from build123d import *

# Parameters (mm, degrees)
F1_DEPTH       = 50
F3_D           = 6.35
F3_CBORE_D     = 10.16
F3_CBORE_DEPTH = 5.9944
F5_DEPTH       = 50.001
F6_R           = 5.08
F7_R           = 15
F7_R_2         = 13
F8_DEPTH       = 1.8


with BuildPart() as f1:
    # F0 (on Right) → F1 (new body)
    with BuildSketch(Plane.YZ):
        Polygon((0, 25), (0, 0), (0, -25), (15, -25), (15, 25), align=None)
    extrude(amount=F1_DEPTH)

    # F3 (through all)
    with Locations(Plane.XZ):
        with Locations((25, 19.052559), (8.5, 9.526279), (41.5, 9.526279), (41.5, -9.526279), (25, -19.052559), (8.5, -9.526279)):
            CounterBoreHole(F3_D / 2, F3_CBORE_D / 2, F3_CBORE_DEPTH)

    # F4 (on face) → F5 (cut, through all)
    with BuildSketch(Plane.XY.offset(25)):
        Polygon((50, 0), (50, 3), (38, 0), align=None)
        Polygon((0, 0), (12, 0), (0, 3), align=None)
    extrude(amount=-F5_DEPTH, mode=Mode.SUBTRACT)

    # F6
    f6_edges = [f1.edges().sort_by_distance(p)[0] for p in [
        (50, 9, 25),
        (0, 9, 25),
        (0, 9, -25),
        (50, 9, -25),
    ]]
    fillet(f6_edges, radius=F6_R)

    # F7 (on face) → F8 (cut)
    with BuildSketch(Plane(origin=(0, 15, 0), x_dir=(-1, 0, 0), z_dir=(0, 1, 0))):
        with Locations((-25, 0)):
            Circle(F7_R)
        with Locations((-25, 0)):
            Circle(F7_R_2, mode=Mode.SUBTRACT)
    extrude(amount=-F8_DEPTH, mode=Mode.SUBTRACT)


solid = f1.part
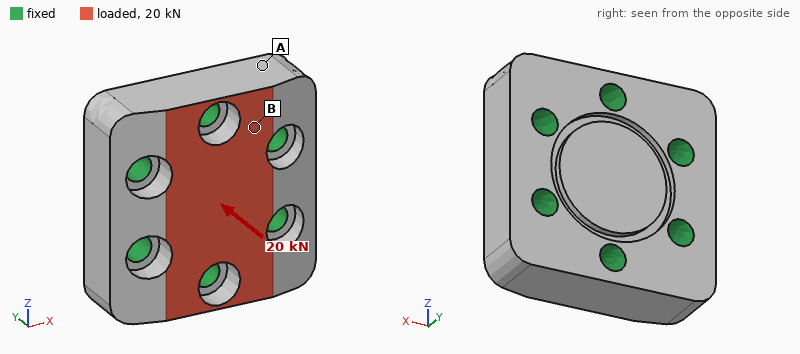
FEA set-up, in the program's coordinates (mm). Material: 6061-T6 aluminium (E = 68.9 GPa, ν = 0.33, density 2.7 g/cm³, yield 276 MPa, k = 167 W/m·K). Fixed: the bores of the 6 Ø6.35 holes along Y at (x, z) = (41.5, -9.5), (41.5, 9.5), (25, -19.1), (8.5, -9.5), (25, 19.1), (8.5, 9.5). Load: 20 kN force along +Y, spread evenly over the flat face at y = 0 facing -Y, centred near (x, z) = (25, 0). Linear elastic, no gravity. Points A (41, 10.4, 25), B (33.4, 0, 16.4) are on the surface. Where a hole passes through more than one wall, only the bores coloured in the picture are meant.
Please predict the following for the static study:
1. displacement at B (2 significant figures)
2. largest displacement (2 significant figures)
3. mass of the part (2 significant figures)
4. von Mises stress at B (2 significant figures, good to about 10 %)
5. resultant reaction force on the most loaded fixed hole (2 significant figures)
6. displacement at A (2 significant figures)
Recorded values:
4.8 µm
8.0 µm
83 g
18 MPa
4.6 kN
3.5 µm
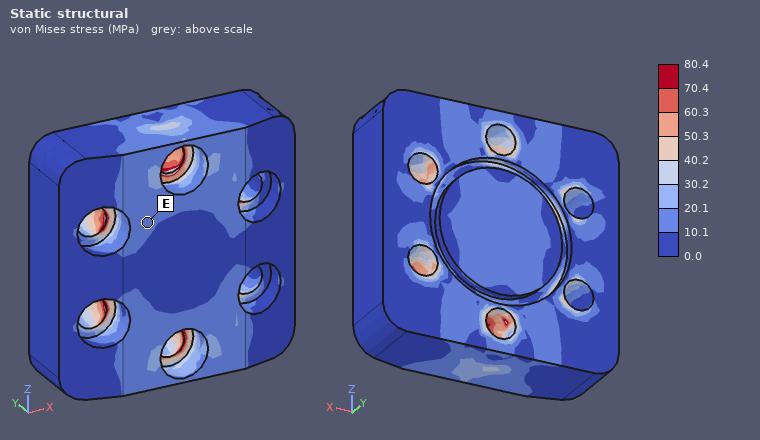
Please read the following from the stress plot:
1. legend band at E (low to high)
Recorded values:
10.1 to 20.1 MPa
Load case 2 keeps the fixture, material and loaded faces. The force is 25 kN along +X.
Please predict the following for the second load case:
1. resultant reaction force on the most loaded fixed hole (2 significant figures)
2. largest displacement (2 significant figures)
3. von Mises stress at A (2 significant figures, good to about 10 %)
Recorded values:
5.4 kN
13 µm
9.1 MPa
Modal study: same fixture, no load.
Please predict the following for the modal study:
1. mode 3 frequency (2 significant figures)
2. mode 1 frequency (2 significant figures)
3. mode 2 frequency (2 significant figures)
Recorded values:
35 kHz
35 kHz
35 kHz
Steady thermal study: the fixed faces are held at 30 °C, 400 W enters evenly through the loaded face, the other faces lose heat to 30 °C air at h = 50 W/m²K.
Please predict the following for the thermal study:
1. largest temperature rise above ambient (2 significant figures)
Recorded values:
30 K
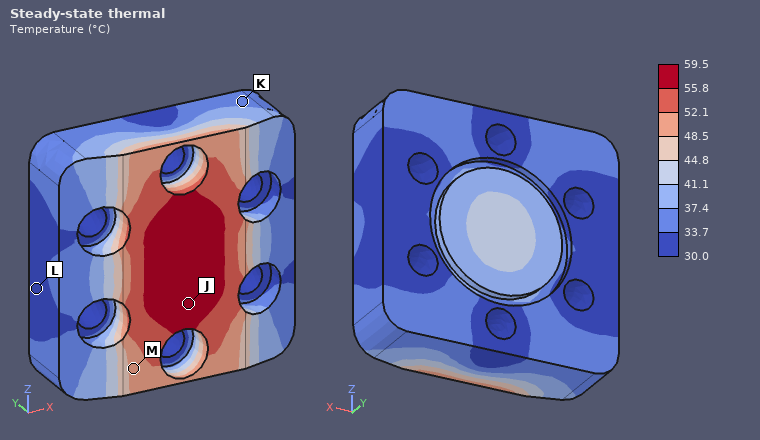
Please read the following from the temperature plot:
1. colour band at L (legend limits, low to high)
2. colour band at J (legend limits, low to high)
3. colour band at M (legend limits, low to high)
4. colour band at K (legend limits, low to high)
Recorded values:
30.0 to 33.7 °C
55.8 to 59.5 °C
48.5 to 52.1 °C
33.7 to 37.4 °C
